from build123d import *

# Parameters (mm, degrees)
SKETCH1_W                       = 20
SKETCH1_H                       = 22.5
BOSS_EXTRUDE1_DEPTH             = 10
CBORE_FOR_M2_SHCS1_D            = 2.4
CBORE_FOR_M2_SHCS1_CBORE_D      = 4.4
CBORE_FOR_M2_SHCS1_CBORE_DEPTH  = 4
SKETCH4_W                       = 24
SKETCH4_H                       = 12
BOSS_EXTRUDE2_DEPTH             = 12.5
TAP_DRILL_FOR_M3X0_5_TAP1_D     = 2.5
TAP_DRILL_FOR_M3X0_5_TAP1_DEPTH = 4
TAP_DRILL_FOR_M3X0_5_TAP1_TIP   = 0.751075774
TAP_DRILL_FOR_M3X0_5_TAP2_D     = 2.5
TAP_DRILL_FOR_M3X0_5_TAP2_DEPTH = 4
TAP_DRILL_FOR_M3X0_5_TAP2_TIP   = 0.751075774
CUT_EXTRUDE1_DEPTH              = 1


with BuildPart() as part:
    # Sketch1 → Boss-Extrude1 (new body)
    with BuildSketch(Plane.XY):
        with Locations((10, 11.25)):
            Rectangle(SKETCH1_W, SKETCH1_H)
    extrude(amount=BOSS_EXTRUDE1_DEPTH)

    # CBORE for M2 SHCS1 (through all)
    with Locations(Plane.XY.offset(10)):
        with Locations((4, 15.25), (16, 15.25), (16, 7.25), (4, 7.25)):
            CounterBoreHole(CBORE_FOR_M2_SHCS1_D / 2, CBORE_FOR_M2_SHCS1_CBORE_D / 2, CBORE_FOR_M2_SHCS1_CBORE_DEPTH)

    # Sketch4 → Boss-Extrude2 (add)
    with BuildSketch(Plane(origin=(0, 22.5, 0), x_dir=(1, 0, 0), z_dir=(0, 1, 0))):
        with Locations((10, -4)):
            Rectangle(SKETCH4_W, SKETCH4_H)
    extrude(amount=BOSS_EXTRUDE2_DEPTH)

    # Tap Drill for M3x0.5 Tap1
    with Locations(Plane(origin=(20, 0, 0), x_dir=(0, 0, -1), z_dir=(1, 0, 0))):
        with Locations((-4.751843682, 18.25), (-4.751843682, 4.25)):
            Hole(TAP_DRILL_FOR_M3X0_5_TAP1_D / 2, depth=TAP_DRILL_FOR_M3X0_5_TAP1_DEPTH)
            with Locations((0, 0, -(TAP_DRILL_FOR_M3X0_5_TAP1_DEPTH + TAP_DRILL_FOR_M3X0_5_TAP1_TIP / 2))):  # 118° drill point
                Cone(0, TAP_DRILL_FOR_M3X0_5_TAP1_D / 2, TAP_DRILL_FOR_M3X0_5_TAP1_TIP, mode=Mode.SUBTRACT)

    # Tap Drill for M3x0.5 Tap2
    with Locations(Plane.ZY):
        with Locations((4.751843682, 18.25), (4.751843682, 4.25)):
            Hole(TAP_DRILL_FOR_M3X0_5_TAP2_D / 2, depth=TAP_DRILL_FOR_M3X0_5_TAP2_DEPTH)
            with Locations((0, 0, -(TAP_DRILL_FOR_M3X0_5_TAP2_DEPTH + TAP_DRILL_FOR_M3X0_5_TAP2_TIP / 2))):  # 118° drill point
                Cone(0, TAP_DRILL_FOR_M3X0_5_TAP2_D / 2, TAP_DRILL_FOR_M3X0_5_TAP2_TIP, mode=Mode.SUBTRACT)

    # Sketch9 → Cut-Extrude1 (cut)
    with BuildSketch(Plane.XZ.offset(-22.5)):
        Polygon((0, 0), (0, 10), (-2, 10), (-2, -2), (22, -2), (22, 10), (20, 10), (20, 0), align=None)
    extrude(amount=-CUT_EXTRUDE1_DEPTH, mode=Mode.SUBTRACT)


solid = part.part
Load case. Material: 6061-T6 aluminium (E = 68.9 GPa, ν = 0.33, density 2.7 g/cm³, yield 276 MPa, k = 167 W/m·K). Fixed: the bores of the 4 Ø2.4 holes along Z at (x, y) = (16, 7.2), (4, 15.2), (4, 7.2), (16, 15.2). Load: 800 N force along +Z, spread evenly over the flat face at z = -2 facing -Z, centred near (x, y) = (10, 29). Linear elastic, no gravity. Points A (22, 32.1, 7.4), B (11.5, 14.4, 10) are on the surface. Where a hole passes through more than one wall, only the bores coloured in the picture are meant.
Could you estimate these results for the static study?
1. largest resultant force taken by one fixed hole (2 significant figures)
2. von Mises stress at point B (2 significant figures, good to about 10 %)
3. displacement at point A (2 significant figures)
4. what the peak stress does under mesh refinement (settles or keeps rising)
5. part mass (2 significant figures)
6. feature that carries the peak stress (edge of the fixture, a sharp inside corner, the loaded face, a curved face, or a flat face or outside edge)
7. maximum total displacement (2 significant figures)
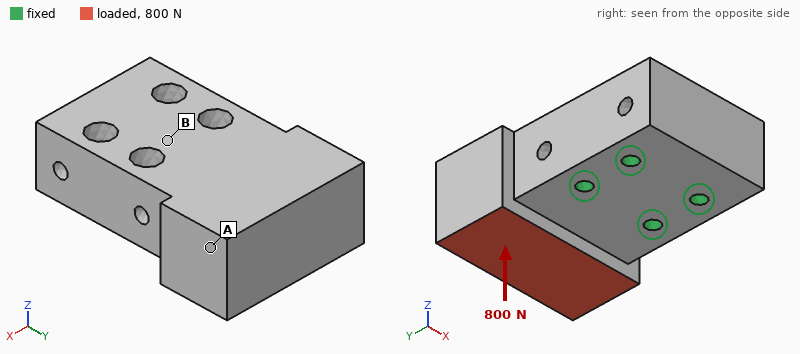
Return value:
720 N
25 MPa
19 µm
keeps rising
20 g
edge of the fixture
24 µm
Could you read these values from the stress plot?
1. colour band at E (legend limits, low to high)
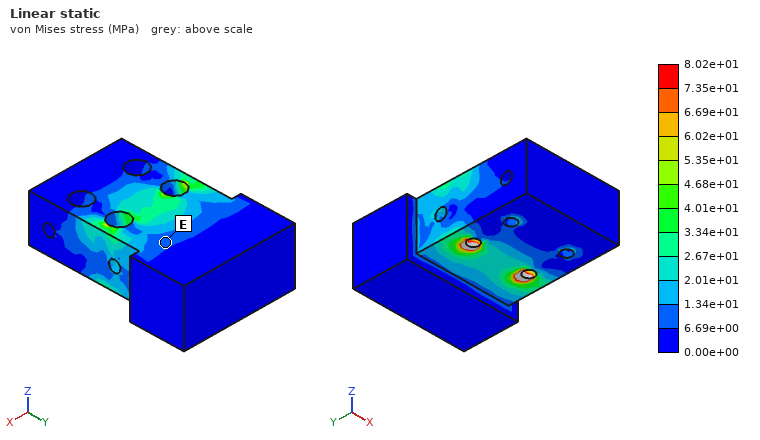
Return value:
6.69e+00 to 1.34e+01 MPa
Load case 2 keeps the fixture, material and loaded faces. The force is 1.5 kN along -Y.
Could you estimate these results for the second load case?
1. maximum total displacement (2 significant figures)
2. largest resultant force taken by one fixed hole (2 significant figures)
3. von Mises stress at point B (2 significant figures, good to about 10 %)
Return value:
24 µm
790 N
17 MPa
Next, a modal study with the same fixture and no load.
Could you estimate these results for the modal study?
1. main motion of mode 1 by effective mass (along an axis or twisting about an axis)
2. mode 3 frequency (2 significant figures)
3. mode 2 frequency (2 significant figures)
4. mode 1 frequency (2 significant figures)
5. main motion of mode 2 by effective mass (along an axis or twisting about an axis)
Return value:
along Z
21 kHz
18 kHz
11 kHz
along X
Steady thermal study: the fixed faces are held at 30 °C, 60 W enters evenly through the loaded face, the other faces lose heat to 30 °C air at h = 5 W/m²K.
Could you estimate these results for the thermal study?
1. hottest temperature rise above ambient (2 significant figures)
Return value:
33 K
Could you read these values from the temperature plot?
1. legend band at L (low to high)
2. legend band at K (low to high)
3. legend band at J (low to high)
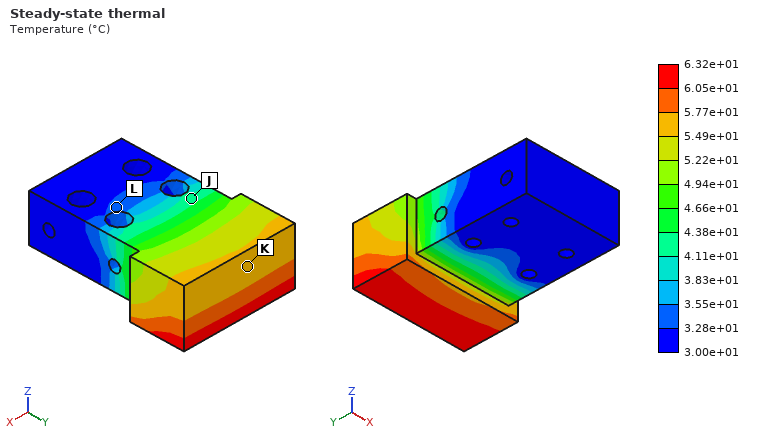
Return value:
3.28e+01 to 3.55e+01 °C
5.49e+01 to 5.77e+01 °C
4.11e+01 to 4.38e+01 °C
